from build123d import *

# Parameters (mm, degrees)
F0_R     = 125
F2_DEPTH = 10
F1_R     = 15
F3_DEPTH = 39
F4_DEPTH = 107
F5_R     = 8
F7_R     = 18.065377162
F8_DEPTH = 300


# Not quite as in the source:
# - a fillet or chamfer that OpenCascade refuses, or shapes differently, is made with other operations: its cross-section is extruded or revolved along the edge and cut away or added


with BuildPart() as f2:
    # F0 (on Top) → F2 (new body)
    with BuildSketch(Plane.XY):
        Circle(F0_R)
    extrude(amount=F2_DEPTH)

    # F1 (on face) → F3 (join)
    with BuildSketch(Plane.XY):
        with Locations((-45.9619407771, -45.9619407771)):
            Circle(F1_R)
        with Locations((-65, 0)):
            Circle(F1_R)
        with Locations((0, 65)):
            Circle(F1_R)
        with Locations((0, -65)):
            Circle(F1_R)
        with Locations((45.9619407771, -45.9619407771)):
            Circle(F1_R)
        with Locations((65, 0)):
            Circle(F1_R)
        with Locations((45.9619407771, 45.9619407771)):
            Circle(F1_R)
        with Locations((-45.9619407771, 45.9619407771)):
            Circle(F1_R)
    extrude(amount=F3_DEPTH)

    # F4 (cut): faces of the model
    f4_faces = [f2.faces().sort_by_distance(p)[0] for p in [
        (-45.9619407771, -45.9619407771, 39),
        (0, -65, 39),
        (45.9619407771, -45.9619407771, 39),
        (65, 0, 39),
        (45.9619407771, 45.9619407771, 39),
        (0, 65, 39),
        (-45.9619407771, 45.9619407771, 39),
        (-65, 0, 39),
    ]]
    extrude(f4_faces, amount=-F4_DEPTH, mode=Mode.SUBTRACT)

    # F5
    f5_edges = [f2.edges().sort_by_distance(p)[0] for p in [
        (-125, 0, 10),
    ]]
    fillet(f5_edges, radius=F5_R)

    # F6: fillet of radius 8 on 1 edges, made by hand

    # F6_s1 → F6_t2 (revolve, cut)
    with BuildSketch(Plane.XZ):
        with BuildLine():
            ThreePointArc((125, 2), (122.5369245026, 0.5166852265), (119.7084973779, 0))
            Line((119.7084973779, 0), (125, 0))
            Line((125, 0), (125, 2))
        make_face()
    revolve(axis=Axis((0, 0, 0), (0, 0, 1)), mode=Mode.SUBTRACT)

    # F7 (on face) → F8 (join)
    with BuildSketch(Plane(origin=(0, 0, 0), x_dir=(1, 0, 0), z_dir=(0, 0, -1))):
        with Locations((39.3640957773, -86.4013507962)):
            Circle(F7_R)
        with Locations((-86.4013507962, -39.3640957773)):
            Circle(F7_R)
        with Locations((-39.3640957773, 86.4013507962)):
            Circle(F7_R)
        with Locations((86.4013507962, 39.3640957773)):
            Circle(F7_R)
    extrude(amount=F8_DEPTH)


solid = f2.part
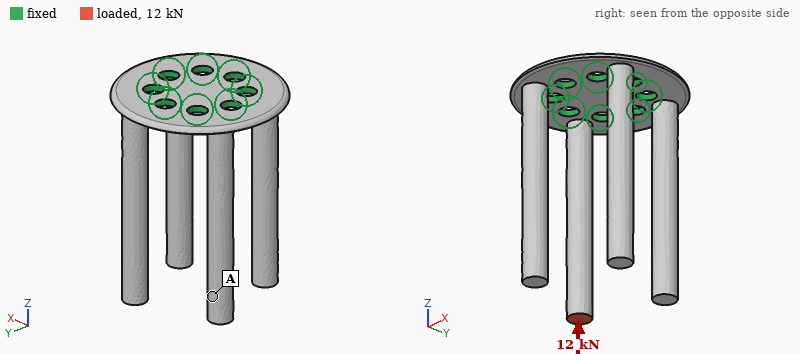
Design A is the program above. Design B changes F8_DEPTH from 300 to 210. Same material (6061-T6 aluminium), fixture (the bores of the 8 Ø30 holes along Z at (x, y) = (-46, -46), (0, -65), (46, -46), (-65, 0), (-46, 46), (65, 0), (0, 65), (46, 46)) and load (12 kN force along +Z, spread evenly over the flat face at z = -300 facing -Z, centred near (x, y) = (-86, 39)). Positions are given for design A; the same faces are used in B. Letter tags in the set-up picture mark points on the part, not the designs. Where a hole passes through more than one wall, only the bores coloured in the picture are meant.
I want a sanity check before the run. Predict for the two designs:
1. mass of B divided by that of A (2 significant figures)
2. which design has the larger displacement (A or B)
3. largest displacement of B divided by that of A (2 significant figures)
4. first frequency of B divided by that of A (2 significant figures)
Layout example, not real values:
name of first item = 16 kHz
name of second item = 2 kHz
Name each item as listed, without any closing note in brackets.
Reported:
mass of B divided by that of A = 0.78
which design has the larger displacement = A
largest displacement of B divided by that of A = 0.72
first frequency of B divided by that of A = 1.8
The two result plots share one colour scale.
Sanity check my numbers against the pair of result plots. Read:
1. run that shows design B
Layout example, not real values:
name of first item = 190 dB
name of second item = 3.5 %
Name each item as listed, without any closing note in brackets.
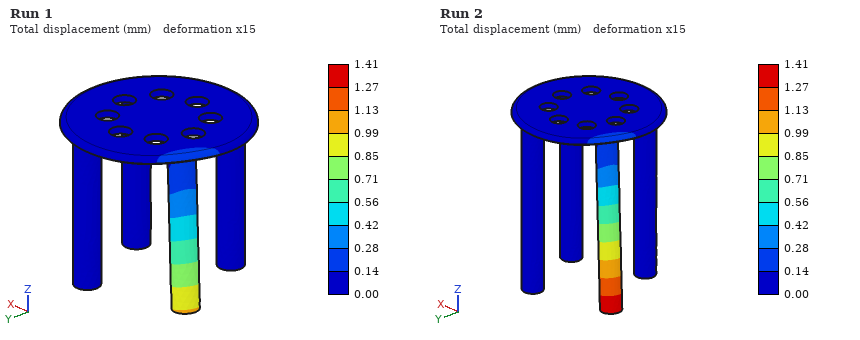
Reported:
run that shows design B = Run 1
